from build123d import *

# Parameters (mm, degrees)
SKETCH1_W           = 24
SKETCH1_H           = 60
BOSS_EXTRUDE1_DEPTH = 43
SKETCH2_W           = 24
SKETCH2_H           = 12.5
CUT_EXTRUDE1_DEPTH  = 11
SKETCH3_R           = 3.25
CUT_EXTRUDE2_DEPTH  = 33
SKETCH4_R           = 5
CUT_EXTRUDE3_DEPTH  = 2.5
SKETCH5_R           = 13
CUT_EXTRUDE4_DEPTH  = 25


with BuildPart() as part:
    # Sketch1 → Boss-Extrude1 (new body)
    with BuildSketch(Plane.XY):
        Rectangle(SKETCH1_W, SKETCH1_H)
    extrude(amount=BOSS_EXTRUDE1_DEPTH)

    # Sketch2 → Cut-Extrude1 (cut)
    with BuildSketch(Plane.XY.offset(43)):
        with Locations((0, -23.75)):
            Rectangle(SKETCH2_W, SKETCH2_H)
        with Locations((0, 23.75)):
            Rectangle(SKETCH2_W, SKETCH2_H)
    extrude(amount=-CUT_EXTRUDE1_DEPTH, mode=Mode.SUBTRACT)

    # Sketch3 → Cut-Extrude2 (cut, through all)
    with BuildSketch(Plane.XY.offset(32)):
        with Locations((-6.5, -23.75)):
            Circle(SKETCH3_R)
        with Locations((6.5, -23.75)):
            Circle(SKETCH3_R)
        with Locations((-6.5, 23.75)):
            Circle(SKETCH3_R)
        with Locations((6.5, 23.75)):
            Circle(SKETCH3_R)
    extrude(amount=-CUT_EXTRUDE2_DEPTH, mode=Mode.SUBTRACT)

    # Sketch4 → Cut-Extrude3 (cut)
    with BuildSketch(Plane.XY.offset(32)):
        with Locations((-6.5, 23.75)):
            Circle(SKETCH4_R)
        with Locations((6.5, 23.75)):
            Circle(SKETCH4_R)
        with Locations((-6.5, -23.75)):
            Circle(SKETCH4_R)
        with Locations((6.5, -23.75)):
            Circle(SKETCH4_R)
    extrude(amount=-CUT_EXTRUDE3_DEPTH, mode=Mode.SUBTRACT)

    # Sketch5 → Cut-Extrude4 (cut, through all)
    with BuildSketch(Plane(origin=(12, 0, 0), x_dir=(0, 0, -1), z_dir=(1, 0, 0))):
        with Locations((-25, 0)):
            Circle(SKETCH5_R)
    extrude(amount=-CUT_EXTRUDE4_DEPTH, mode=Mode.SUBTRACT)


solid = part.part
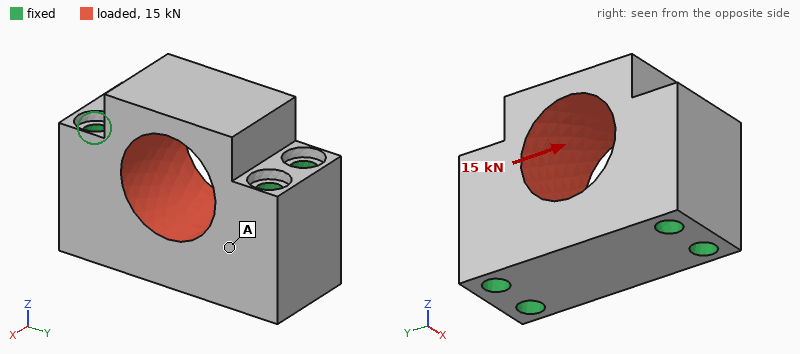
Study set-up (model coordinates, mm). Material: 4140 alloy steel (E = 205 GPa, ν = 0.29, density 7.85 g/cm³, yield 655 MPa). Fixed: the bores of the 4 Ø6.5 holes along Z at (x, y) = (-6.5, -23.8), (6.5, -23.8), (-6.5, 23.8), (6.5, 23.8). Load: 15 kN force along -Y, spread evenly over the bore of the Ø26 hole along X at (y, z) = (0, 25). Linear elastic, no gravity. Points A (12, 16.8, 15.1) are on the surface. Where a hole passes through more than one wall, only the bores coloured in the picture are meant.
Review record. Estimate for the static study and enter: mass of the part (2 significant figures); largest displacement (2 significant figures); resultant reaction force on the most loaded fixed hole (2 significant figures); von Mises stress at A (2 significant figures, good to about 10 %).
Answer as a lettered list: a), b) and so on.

a) 300 g
b) 5.5 µm
c) 3.9 kN
d) 6.6 MPa
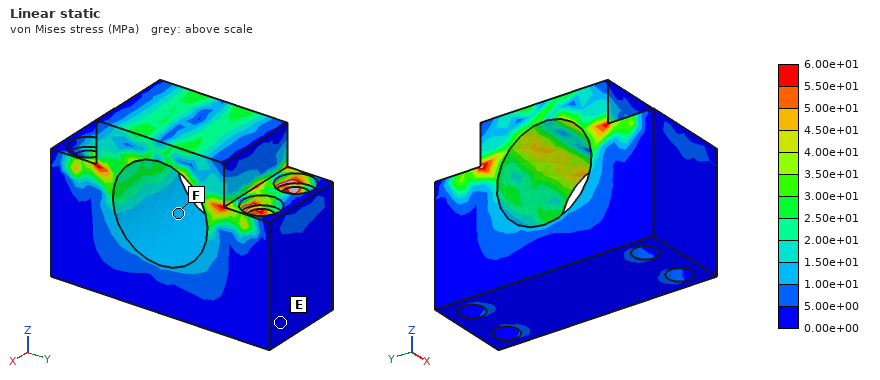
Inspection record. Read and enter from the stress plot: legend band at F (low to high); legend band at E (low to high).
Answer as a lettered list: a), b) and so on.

a) 1.00e+01 to 1.50e+01 MPa
b) 0.00e+00 to 5.00e+00 MPa
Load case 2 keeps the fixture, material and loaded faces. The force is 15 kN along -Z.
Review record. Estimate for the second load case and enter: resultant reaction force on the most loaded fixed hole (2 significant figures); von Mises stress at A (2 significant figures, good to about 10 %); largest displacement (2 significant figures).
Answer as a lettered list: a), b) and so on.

a) 3.8 kN
b) 16 MPa
c) 4.8 µm
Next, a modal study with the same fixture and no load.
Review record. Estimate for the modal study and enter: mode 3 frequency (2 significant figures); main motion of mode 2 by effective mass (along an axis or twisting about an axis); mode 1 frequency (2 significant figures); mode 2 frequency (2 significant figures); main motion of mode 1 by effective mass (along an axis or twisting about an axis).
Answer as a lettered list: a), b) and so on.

a) 26 kHz
b) along Y
c) 19 kHz
d) 22 kHz
e) along X
